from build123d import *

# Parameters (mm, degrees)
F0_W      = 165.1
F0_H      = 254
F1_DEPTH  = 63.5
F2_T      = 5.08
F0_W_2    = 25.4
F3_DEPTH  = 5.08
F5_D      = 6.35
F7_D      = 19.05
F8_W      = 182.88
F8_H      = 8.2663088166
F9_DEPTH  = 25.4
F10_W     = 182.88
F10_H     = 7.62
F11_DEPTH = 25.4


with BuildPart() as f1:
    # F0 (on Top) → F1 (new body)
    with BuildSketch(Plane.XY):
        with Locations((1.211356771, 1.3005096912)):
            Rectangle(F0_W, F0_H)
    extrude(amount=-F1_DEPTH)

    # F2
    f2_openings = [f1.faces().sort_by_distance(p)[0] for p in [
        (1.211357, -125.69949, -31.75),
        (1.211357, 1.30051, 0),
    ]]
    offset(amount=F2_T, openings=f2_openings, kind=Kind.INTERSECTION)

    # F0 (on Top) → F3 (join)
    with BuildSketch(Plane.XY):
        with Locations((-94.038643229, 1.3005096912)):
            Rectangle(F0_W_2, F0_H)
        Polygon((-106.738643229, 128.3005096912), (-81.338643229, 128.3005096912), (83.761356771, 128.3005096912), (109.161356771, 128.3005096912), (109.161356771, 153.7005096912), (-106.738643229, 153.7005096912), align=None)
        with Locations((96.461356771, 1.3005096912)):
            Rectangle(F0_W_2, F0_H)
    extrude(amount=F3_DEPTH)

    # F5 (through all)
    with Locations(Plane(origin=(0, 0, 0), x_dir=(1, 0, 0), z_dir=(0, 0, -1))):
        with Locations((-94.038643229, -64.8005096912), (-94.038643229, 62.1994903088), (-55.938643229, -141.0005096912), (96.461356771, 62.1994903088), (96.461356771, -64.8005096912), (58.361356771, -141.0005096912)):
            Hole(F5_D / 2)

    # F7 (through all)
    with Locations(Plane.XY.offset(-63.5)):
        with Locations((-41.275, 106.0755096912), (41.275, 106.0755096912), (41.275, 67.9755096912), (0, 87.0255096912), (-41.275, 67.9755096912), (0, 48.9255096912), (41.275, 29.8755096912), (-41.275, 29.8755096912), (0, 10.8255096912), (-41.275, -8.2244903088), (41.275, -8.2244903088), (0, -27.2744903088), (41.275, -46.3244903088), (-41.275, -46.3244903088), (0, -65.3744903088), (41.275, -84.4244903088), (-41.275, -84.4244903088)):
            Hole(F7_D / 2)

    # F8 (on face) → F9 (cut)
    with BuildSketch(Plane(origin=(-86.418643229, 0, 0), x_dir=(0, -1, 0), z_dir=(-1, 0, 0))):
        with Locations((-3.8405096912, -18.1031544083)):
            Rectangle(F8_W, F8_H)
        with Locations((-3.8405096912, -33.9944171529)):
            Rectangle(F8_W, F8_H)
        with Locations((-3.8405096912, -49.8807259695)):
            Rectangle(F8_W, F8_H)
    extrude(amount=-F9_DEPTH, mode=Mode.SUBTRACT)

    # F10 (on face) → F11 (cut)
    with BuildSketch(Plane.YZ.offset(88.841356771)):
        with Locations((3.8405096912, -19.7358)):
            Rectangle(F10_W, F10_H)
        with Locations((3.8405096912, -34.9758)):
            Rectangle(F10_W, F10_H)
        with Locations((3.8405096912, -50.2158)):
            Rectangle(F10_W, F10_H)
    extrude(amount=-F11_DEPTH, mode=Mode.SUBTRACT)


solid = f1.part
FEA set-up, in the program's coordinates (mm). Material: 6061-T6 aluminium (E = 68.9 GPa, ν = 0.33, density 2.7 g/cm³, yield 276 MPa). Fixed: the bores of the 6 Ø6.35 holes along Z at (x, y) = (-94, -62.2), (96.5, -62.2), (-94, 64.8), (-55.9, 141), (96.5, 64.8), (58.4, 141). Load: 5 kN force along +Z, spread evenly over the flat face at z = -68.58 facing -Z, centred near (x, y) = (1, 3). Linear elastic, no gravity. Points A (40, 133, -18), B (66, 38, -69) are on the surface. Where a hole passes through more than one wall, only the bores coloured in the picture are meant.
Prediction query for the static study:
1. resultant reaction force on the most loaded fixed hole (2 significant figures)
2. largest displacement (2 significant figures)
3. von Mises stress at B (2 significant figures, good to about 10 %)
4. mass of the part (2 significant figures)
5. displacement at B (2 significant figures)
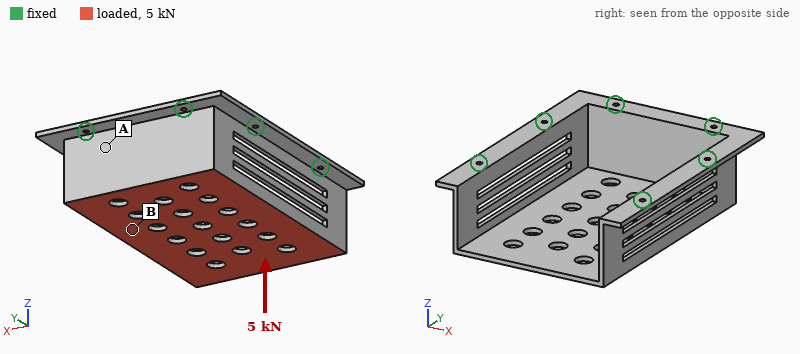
1.6 kN
1.2 mm
31 MPa
1.3 kg
0.50 mm
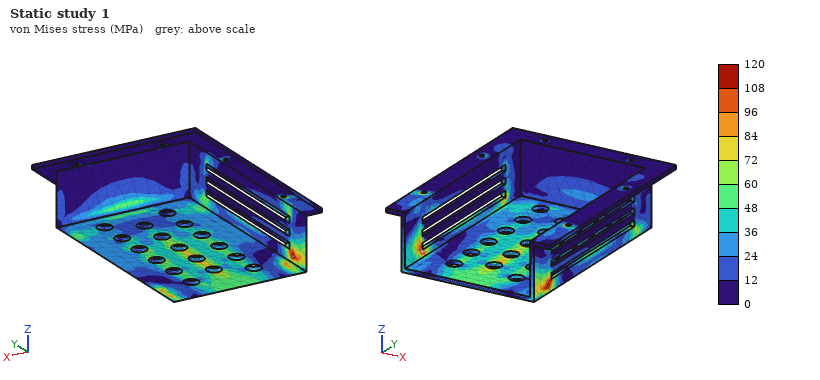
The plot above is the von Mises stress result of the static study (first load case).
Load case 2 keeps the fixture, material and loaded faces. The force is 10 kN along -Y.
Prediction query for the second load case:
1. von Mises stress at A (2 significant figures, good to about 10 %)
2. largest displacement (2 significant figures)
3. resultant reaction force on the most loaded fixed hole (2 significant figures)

29 MPa
0.49 mm
5.5 kN
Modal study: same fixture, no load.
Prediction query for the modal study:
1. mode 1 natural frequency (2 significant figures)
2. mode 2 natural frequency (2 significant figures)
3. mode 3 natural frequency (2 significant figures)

520 Hz
530 Hz
650 Hz
